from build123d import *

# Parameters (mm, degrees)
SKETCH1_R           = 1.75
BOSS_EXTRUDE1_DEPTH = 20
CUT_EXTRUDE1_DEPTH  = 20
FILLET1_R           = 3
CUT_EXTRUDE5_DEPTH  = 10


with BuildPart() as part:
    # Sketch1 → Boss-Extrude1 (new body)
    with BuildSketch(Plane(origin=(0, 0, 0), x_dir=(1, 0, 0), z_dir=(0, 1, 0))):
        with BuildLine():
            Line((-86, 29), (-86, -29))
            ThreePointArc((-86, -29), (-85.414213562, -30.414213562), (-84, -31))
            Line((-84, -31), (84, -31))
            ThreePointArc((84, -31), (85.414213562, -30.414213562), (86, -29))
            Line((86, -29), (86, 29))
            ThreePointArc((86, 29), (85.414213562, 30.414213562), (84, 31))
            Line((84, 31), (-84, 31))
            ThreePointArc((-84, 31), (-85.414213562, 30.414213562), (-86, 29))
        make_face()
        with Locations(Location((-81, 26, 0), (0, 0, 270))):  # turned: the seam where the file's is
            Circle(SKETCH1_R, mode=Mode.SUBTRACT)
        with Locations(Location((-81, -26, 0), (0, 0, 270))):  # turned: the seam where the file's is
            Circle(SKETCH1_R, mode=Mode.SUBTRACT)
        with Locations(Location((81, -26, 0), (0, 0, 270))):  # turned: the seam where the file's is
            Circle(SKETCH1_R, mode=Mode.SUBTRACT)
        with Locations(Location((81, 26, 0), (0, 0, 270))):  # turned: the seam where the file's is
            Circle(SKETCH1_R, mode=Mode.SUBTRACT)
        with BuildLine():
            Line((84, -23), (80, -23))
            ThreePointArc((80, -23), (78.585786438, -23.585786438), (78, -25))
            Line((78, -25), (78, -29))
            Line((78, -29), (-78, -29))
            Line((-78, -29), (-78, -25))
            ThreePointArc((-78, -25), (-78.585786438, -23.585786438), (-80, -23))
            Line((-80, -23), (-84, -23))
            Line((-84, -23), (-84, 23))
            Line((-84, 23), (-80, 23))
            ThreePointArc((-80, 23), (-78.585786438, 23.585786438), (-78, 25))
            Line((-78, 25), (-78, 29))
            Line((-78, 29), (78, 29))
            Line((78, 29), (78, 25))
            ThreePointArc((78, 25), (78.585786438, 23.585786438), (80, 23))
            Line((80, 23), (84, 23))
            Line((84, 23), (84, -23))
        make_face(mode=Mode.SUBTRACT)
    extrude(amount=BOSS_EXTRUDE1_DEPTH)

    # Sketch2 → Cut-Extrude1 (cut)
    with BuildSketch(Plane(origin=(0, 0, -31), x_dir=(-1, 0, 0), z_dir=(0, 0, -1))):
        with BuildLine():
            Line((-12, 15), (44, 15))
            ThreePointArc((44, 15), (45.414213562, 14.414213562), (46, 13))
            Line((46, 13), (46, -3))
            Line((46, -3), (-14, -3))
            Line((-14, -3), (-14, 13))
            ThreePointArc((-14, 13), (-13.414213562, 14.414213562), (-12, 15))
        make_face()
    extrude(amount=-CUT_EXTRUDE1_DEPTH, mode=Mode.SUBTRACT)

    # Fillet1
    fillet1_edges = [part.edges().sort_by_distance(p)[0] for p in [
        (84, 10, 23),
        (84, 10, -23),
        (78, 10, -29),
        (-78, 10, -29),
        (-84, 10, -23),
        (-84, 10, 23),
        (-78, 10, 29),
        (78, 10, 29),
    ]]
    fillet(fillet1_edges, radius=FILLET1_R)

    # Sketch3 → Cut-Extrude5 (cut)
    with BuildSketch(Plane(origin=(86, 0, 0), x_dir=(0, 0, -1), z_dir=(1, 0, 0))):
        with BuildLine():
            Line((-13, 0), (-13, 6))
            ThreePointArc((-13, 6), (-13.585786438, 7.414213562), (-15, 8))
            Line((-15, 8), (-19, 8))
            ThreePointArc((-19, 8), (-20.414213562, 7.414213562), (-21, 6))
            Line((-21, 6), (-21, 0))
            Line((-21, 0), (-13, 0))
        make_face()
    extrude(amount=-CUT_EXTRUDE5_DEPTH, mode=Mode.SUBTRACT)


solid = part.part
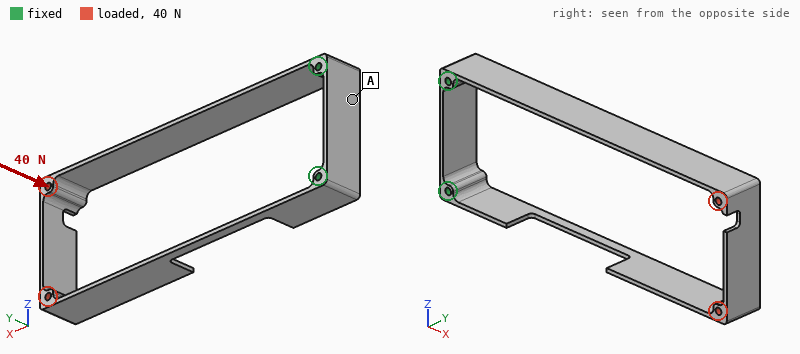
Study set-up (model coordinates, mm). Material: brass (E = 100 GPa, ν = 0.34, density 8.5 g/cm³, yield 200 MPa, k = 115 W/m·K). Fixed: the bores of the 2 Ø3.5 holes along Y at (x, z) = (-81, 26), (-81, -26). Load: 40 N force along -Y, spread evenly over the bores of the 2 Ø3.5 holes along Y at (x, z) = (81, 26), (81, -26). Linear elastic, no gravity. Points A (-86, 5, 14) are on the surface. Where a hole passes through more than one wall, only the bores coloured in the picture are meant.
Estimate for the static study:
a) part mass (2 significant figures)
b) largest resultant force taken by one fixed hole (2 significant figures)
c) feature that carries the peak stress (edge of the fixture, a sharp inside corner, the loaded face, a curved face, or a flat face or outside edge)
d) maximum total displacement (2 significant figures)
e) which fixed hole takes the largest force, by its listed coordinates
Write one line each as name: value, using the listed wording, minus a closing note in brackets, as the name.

part mass: 160 g
largest resultant force taken by one fixed hole: 31 N
feature that carries the peak stress: a curved face
maximum total displacement: 2.0 mm
which fixed hole takes the largest force, by its listed coordinates: (-81, 26)
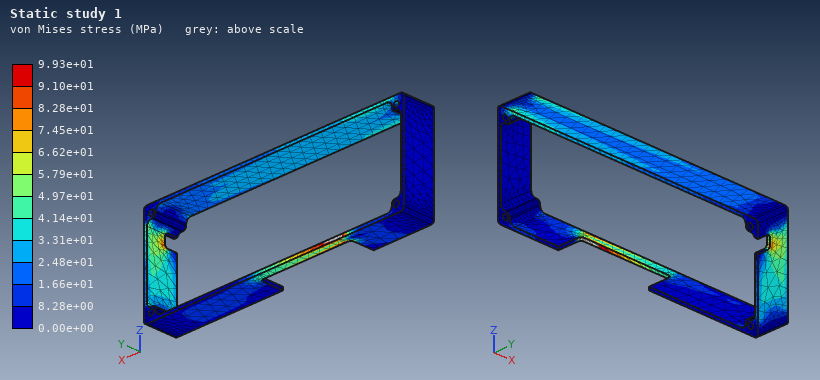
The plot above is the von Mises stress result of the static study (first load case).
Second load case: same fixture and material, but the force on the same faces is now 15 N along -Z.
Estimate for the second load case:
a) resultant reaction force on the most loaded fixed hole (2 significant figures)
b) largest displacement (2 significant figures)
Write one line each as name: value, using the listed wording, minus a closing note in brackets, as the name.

resultant reaction force on the most loaded fixed hole: 23 N
largest displacement: 2.2 mm
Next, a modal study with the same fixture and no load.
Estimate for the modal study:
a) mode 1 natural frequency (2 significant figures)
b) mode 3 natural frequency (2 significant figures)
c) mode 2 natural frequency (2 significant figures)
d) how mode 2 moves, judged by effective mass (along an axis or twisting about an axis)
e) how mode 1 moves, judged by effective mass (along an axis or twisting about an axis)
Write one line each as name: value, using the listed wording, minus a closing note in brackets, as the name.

mode 1 natural frequency: 50 Hz
mode 3 natural frequency: 230 Hz
mode 2 natural frequency: 100 Hz
how mode 2 moves, judged by effective mass: along Y
how mode 1 moves, judged by effective mass: along Z
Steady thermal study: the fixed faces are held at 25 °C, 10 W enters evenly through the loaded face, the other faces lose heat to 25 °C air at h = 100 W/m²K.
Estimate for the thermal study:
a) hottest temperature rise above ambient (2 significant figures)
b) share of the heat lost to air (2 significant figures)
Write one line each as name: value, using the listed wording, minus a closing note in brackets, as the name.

hottest temperature rise above ambient: 19 K
share of the heat lost to air: 99 %
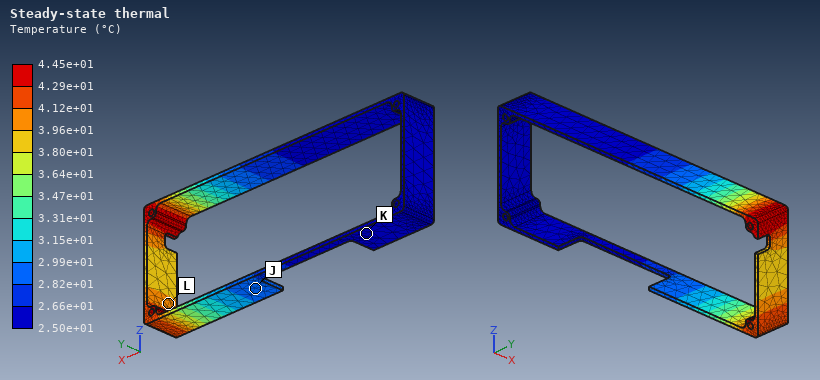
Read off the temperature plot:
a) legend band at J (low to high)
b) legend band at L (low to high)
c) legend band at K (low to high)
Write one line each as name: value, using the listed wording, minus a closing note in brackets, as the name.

legend band at J: 2.82e+01 to 2.99e+01 °C
legend band at L: 3.96e+01 to 4.12e+01 °C
legend band at K: 2.50e+01 to 2.66e+01 °C
